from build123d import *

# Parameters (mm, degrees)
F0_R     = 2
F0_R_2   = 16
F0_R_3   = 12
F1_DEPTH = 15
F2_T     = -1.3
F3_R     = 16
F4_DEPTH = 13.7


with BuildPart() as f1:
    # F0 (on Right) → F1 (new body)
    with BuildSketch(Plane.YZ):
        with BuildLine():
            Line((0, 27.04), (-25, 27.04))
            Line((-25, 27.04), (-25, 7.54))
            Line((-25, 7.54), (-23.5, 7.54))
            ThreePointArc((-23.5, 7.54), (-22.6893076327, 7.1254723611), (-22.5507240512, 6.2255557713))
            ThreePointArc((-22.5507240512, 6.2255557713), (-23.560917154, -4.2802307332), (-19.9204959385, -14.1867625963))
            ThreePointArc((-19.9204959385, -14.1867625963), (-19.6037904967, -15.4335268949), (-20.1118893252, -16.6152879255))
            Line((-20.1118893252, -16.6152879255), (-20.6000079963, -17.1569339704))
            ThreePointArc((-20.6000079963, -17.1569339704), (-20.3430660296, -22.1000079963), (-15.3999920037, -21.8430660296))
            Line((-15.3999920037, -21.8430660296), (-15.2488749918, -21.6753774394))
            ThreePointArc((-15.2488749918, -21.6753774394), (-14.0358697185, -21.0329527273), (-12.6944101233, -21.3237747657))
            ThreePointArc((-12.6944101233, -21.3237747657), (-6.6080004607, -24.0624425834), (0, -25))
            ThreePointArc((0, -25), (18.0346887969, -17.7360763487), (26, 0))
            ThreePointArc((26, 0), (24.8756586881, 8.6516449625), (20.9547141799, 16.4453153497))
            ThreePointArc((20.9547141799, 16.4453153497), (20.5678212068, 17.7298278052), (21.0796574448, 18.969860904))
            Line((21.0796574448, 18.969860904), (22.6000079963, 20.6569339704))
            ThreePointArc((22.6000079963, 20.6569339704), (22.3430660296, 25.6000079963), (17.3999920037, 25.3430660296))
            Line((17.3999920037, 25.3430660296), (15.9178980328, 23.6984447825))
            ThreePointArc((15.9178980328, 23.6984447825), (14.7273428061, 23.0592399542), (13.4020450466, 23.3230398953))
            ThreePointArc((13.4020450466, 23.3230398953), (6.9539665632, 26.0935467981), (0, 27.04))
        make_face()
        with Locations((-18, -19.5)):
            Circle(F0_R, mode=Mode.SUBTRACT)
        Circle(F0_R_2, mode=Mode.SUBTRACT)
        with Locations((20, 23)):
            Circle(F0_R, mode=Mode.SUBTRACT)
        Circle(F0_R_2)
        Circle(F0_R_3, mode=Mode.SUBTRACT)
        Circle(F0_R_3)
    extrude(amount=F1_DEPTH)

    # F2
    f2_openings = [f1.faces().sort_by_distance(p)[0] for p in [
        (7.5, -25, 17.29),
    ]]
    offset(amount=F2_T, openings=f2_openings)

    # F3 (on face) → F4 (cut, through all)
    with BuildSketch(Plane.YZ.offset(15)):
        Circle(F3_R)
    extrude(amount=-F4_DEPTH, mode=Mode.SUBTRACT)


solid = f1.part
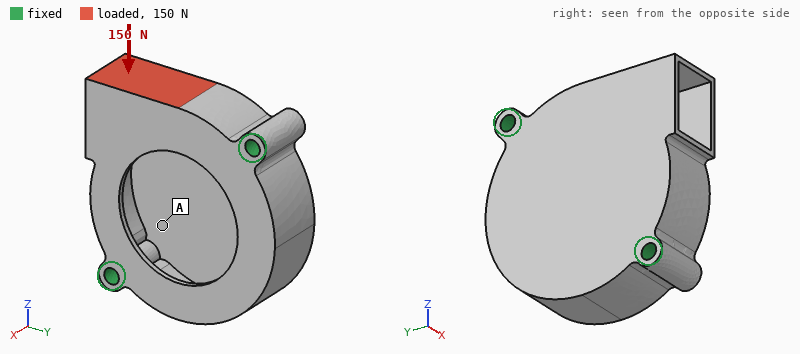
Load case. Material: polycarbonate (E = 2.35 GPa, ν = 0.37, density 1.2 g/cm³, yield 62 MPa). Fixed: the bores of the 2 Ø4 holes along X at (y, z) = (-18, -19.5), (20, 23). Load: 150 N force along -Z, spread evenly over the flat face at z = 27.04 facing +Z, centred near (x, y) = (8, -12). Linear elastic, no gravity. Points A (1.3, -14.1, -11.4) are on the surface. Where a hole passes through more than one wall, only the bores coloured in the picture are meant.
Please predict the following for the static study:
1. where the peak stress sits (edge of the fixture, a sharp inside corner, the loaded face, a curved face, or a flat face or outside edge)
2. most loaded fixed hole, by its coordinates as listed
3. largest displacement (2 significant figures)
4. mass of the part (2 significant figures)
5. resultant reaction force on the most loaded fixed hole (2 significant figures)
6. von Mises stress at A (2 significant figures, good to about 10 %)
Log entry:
the loaded face
(-18, -19.5)
0.31 mm
9.3 g
110 N
2.5 MPa
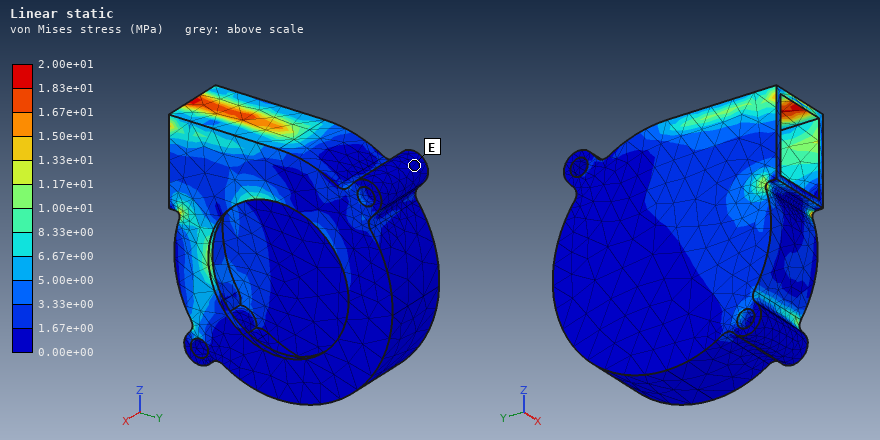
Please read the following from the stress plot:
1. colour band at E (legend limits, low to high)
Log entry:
0.00e+00 to 1.67e+00 MPa
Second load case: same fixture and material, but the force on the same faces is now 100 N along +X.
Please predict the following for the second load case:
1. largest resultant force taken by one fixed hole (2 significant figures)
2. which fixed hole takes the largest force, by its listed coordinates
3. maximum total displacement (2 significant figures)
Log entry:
95 N
(20, 23)
0.80 mm
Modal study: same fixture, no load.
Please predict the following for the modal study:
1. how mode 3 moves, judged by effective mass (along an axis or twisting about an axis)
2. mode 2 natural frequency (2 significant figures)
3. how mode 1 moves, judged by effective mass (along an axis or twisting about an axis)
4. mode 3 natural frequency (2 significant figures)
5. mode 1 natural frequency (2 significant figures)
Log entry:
along X
1700 Hz
along X
2200 Hz
1300 Hz
